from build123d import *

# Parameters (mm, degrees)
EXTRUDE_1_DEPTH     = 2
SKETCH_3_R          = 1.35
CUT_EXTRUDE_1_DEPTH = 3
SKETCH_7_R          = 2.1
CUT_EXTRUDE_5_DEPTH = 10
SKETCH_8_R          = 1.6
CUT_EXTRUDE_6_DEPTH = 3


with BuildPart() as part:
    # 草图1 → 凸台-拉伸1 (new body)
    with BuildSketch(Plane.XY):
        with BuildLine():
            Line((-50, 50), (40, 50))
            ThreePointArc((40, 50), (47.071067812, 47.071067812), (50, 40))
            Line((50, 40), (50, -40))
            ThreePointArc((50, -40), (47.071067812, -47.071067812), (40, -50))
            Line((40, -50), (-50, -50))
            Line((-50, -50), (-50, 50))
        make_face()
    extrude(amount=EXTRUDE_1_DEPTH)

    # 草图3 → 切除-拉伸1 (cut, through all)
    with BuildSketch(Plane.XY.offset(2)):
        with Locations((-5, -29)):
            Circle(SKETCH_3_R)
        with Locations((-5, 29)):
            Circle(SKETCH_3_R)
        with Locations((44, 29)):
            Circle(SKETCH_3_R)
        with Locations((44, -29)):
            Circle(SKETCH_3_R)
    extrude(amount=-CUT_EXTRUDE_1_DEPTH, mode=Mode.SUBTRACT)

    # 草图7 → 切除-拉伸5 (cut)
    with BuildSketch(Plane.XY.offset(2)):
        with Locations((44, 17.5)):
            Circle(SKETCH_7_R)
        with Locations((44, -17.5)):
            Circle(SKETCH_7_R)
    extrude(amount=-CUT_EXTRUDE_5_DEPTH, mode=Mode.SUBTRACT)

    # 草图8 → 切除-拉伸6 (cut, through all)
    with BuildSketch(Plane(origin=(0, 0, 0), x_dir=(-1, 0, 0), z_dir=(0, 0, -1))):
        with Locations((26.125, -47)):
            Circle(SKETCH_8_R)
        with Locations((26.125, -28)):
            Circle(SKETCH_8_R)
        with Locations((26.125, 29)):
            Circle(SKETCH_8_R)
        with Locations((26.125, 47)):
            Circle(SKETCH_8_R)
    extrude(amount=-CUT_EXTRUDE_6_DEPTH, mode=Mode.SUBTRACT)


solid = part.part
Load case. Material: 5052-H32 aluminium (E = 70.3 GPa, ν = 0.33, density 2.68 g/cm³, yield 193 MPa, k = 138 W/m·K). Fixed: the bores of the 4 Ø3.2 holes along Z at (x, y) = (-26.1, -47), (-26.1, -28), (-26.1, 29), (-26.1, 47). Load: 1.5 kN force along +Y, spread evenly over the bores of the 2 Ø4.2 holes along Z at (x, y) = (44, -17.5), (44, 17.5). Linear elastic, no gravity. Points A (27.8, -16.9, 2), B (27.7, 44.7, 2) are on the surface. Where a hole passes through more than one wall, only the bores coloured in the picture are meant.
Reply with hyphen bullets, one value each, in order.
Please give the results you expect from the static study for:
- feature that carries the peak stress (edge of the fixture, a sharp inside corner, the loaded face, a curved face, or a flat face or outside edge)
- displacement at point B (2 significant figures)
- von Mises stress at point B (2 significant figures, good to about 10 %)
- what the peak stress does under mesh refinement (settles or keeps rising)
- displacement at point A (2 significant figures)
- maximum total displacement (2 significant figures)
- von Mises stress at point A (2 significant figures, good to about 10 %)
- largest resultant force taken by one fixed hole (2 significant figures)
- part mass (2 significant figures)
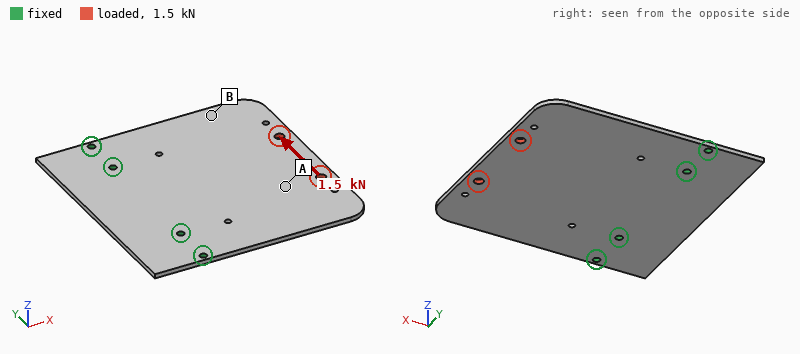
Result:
- edge of the fixture
- 33 µm
- 7.2 MPa
- keeps rising
- 29 µm
- 44 µm
- 17 MPa
- 850 N
- 53 g
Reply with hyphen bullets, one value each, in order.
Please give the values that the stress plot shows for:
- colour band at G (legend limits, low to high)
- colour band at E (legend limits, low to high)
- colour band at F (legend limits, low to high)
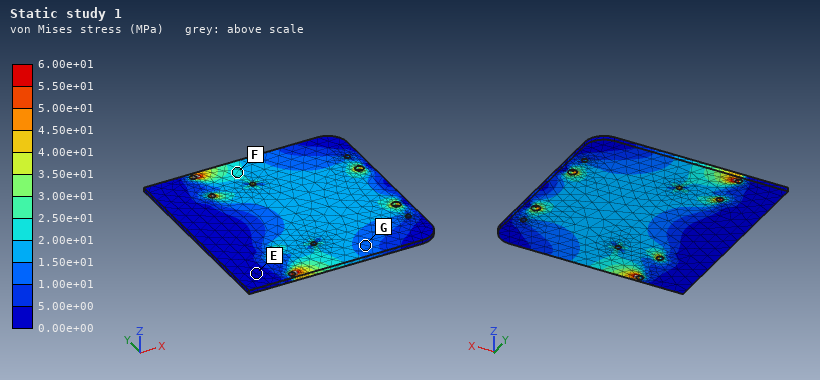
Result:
- 1.00e+01 to 1.50e+01 MPa
- 0.00e+00 to 5.00e+00 MPa
- 2.00e+01 to 2.50e+01 MPa
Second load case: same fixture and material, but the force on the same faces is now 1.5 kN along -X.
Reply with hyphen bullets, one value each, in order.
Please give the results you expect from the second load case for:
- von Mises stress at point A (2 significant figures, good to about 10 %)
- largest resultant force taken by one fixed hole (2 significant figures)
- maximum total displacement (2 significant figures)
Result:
- 13 MPa
- 510 N
- 15 µm
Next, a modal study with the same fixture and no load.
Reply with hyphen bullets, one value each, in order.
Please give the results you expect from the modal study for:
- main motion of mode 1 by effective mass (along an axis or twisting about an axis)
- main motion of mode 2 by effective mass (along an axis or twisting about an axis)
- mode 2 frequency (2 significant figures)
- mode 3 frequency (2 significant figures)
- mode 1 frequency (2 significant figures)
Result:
- along Z
- twisting about X
- 600 Hz
- 1500 Hz
- 280 Hz
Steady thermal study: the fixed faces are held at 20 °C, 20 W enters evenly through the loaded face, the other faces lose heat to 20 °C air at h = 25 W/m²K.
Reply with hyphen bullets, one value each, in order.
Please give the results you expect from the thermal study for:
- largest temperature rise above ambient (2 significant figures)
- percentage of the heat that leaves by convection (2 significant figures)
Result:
- 52 K
- 43 %
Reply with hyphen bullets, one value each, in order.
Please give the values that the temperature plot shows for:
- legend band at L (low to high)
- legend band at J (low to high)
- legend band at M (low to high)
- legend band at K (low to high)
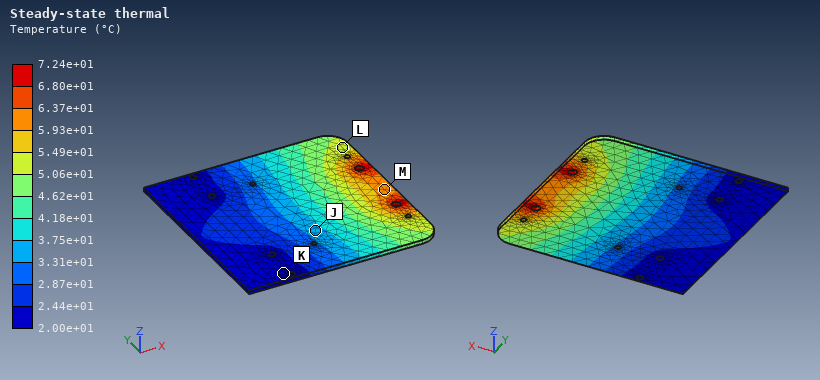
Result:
- 5.06e+01 to 5.49e+01 °C
- 3.31e+01 to 3.75e+01 °C
- 5.93e+01 to 6.37e+01 °C
- 2.00e+01 to 2.44e+01 °C
